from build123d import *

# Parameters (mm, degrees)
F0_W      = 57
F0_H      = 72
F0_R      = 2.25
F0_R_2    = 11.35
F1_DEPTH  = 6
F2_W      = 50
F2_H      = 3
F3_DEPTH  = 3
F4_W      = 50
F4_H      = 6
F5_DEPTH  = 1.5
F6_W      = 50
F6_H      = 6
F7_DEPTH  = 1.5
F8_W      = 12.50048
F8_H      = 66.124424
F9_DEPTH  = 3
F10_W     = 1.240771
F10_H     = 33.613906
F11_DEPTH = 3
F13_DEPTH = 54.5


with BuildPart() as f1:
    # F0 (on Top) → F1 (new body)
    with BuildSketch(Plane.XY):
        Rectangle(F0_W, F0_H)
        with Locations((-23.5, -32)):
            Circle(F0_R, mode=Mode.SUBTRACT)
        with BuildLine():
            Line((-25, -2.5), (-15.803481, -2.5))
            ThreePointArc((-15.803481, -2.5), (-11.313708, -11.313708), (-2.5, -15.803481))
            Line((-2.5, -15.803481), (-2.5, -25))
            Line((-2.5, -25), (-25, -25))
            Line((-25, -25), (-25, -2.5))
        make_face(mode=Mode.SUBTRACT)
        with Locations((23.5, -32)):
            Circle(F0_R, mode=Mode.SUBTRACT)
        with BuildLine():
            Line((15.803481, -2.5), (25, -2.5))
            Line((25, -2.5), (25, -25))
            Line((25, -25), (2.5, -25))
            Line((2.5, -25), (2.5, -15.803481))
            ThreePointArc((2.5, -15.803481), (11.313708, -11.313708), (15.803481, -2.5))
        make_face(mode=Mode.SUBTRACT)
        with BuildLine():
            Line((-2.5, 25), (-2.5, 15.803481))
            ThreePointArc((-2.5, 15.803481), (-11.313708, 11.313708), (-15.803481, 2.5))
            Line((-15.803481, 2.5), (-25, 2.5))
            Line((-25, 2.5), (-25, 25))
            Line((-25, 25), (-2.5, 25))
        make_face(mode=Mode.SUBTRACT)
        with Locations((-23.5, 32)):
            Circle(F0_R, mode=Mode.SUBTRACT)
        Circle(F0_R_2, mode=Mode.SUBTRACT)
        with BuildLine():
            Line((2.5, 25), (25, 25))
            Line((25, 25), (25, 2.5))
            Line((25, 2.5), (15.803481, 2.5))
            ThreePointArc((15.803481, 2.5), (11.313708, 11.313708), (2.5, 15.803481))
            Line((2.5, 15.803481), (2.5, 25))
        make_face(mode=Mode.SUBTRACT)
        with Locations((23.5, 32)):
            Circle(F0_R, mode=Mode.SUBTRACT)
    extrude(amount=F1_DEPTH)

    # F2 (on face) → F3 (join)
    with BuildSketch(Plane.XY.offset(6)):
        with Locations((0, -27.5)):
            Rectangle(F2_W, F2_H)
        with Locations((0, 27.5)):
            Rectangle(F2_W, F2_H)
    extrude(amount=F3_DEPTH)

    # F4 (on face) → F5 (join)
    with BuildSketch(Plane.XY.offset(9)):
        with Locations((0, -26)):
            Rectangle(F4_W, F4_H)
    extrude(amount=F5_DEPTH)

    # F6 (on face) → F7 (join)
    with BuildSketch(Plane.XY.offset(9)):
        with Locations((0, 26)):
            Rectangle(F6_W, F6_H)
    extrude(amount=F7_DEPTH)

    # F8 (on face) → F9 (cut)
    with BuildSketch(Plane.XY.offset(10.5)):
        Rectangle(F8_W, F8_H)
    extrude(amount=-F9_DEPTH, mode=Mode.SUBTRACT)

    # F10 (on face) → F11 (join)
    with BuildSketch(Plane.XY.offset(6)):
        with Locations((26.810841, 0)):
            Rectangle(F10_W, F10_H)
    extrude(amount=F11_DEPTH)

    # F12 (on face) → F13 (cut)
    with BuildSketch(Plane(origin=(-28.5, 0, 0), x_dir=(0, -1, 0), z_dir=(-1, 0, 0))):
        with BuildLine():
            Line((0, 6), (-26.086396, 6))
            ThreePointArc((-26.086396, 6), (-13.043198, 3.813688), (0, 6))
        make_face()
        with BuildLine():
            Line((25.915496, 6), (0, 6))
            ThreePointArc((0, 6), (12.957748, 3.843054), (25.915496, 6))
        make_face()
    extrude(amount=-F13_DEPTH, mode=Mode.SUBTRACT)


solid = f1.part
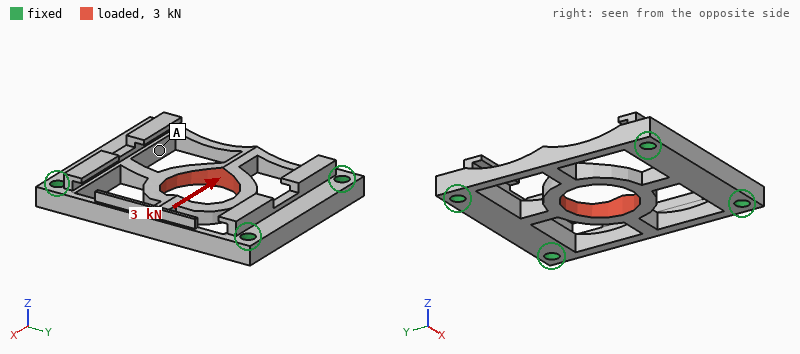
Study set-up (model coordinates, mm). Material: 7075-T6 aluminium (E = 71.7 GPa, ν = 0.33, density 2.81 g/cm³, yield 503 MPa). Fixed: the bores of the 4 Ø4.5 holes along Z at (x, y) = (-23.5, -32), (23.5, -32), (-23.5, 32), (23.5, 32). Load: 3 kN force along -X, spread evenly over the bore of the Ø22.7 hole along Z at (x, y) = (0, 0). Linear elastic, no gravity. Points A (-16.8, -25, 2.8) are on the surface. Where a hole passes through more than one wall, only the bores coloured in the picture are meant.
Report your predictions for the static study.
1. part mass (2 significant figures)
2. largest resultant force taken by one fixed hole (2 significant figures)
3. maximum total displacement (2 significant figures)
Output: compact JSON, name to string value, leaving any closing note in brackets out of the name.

{"part mass": "37 g", "largest resultant force taken by one fixed hole": "860 N", "maximum total displacement": "0.12 mm"}
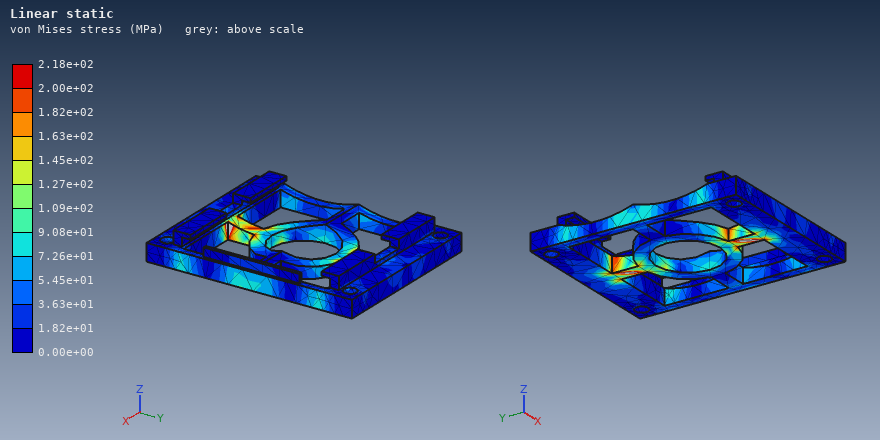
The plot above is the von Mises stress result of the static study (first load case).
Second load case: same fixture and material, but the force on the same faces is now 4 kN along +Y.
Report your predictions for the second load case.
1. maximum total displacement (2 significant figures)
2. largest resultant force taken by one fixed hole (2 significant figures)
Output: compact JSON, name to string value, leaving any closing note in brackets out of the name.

{"maximum total displacement": "86 µm", "largest resultant force taken by one fixed hole": "1.1 kN"}
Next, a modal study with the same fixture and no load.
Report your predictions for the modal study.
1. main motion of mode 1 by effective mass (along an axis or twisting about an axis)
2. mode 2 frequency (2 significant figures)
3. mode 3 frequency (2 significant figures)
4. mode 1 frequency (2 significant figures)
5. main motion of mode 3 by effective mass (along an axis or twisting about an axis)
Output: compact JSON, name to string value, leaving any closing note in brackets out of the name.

{"main motion of mode 1 by effective mass": "along Z", "mode 2 frequency": "6800 Hz", "mode 3 frequency": "8800 Hz", "mode 1 frequency": "5400 Hz", "main motion of mode 3 by effective mass": "along X"}
